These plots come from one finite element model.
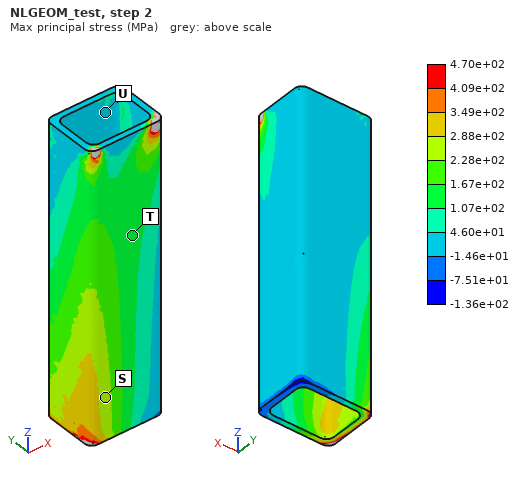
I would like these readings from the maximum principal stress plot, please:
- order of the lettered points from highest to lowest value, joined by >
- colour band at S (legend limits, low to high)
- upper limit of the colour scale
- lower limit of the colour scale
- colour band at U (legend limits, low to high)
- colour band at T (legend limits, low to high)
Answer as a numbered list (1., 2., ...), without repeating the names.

1. S > T > U
2. 2.28e+02 to 2.88e+02 MPa
3. 4.70e+02 MPa
4. -1.36e+02 MPa
5. -1.46e+01 to 4.60e+01 MPa
6. 1.07e+02 to 1.67e+02 MPa
